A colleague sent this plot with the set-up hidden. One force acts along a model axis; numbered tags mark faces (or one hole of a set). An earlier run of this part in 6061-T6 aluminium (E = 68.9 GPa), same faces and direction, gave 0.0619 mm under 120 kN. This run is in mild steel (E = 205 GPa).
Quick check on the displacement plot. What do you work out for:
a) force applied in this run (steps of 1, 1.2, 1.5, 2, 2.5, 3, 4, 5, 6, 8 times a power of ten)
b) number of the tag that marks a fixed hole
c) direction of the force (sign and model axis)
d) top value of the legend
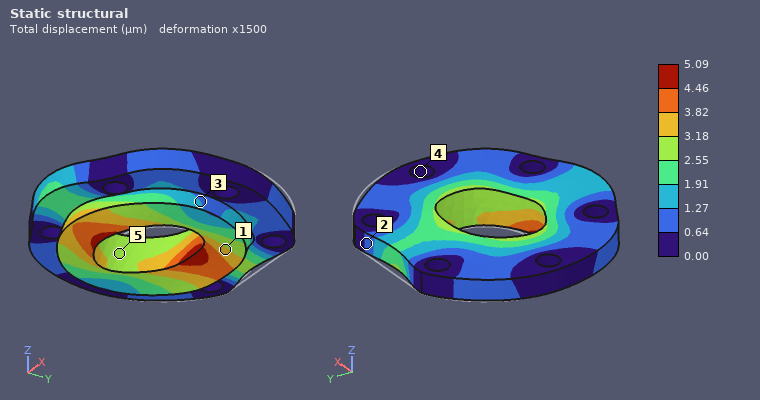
30 kN
4
-Y
5.09 µm
